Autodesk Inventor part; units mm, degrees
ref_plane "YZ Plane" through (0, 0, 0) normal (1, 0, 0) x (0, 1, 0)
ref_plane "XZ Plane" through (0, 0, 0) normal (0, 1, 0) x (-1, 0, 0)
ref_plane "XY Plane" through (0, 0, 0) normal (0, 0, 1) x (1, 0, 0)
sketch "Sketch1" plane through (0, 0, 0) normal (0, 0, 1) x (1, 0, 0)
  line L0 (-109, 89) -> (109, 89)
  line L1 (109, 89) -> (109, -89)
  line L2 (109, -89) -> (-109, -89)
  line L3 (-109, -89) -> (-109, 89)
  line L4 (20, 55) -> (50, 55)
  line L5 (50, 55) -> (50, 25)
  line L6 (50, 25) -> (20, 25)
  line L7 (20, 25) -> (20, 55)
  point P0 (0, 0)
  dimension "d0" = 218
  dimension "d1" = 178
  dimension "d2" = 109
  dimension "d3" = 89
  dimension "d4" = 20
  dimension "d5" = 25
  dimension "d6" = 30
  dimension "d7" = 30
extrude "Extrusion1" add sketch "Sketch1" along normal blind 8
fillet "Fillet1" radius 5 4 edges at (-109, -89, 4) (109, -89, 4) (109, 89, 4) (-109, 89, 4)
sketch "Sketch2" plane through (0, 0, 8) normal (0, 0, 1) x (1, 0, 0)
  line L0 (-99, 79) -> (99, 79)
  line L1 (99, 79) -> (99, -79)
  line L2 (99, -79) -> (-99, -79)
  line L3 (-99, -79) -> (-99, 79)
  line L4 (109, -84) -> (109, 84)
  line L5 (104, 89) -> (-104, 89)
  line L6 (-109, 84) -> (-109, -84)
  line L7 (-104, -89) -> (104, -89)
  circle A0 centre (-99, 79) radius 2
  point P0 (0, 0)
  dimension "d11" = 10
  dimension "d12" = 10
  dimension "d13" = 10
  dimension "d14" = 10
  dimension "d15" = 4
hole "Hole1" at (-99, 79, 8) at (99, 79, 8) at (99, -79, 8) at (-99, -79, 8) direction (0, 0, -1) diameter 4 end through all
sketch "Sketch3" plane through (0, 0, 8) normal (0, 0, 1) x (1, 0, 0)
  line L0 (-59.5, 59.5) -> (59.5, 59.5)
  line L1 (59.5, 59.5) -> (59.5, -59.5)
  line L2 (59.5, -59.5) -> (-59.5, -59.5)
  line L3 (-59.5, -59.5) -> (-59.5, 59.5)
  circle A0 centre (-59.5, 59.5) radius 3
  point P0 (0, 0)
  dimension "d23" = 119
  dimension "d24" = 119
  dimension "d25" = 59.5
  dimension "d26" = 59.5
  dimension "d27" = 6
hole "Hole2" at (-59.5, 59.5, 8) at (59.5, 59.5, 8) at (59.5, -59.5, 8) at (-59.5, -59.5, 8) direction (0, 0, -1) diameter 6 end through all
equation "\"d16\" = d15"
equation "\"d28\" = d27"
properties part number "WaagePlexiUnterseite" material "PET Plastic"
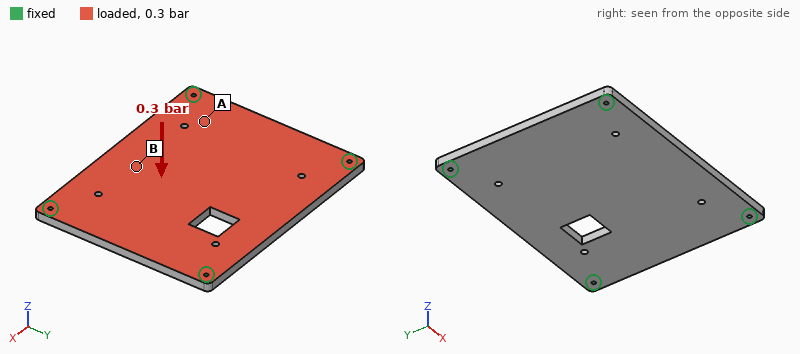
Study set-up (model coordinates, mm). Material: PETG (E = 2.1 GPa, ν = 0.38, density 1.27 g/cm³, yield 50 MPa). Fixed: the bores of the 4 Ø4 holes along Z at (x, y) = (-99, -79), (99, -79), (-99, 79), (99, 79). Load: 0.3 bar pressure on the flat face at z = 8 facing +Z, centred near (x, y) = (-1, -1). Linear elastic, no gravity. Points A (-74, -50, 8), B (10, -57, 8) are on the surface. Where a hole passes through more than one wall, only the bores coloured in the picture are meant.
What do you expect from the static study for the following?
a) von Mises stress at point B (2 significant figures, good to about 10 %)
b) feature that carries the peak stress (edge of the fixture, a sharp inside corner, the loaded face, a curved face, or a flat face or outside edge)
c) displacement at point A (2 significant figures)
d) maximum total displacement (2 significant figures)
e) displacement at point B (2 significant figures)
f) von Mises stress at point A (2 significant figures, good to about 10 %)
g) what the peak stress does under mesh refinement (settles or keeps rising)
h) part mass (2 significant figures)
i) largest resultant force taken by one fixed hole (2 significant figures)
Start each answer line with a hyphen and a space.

- 6.2 MPa
- edge of the fixture
- 1.2 mm
- 3.2 mm
- 2.7 mm
- 2.0 MPa
- keeps rising
- 380 g
- 290 N
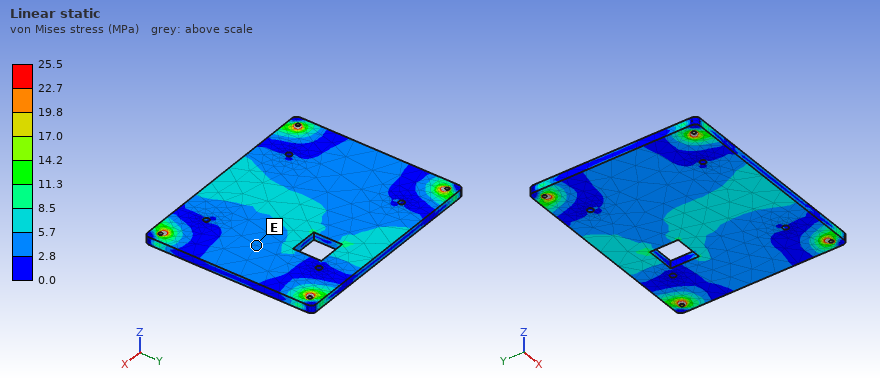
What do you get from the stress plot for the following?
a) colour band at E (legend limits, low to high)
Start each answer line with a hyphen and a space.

- 2.8 to 5.7 MPa
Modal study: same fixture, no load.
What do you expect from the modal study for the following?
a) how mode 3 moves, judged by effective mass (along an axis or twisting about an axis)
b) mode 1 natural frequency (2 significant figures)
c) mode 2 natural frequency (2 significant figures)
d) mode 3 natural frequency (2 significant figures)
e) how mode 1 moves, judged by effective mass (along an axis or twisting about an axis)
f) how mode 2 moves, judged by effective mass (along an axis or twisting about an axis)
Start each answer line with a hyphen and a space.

- twisting about Y
- 180 Hz
- 300 Hz
- 380 Hz
- along Z
- twisting about X
